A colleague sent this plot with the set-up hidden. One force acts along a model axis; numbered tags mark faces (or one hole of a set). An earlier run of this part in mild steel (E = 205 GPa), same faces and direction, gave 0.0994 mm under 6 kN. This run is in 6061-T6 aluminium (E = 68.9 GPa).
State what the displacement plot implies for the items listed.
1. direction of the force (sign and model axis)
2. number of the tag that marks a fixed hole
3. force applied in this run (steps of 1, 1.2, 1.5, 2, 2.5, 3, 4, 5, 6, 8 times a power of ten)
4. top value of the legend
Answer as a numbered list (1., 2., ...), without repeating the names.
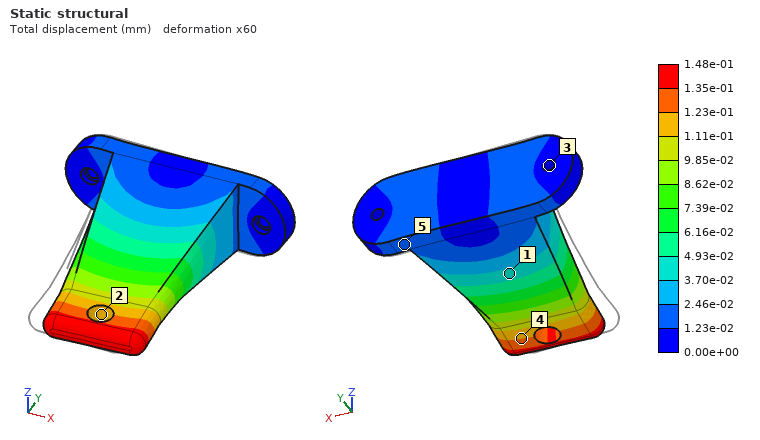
1. +X
2. 3
3. 3 kN
4. 1.48e-01 mm
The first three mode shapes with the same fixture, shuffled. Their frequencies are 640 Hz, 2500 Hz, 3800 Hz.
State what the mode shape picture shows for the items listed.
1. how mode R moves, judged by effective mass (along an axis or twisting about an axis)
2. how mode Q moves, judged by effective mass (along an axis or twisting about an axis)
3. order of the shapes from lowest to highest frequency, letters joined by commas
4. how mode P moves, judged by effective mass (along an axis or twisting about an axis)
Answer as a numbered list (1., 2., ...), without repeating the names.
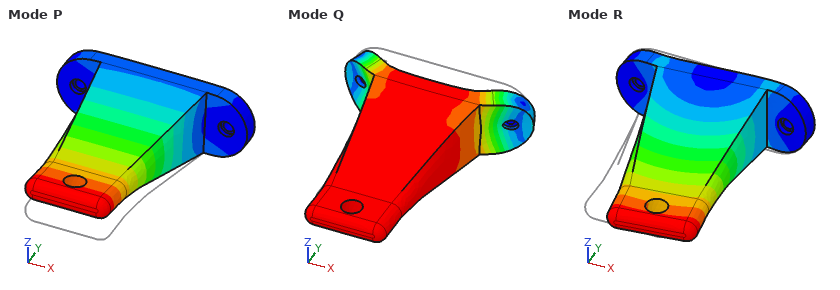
1. along X
2. along Y
3. P, R, Q
4. along Z
